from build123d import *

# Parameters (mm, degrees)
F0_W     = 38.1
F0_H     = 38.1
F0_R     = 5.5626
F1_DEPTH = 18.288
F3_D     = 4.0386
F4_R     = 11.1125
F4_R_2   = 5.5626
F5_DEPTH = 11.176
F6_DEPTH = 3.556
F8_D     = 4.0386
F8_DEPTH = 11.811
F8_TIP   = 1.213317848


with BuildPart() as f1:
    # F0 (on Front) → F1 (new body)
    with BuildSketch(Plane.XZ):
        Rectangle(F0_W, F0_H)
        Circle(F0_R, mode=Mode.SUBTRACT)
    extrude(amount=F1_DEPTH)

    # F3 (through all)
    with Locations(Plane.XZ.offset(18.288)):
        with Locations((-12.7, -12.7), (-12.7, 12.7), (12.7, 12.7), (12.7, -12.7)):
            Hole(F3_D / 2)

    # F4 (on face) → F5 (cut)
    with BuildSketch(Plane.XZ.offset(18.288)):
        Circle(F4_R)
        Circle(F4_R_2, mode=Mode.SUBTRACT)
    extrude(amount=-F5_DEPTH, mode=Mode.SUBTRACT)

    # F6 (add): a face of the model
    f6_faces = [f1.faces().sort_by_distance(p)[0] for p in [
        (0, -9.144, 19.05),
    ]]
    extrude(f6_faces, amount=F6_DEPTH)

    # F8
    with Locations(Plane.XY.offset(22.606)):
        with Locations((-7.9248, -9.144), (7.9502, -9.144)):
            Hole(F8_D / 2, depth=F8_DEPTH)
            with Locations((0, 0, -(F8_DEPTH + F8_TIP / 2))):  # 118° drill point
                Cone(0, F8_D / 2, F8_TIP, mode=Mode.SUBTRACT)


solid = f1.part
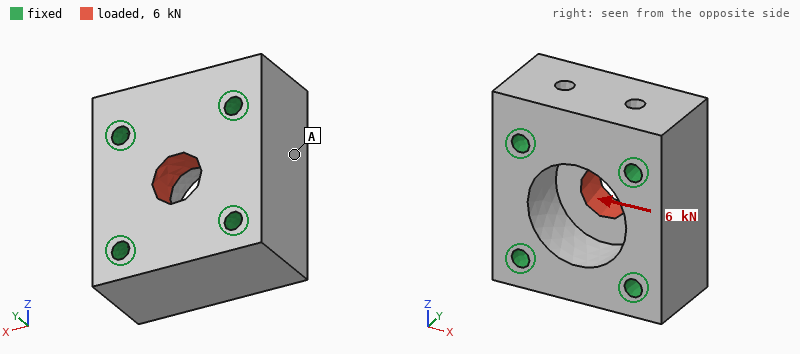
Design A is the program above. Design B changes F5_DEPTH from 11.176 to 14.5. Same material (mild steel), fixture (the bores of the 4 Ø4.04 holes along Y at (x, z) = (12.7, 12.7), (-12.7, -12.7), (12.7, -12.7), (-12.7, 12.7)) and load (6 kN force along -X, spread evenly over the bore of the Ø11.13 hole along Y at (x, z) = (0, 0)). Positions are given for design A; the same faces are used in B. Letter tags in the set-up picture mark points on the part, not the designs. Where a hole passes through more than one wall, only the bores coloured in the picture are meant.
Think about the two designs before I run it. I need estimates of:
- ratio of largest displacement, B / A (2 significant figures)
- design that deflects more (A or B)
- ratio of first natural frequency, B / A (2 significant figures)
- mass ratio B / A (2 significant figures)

1.7
B
0.99
0.96
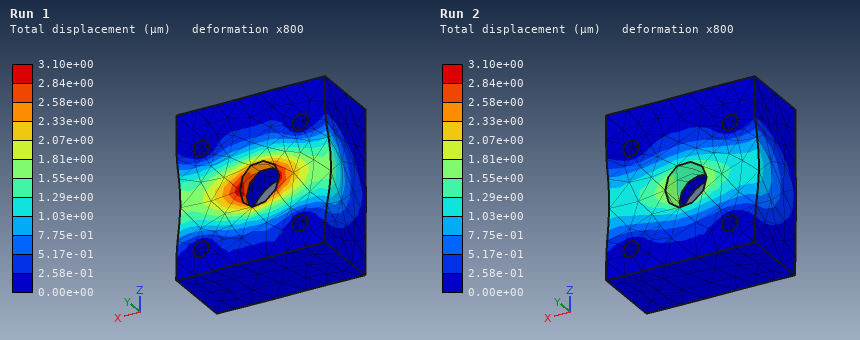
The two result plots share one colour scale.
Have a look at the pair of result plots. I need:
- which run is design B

Run 1
